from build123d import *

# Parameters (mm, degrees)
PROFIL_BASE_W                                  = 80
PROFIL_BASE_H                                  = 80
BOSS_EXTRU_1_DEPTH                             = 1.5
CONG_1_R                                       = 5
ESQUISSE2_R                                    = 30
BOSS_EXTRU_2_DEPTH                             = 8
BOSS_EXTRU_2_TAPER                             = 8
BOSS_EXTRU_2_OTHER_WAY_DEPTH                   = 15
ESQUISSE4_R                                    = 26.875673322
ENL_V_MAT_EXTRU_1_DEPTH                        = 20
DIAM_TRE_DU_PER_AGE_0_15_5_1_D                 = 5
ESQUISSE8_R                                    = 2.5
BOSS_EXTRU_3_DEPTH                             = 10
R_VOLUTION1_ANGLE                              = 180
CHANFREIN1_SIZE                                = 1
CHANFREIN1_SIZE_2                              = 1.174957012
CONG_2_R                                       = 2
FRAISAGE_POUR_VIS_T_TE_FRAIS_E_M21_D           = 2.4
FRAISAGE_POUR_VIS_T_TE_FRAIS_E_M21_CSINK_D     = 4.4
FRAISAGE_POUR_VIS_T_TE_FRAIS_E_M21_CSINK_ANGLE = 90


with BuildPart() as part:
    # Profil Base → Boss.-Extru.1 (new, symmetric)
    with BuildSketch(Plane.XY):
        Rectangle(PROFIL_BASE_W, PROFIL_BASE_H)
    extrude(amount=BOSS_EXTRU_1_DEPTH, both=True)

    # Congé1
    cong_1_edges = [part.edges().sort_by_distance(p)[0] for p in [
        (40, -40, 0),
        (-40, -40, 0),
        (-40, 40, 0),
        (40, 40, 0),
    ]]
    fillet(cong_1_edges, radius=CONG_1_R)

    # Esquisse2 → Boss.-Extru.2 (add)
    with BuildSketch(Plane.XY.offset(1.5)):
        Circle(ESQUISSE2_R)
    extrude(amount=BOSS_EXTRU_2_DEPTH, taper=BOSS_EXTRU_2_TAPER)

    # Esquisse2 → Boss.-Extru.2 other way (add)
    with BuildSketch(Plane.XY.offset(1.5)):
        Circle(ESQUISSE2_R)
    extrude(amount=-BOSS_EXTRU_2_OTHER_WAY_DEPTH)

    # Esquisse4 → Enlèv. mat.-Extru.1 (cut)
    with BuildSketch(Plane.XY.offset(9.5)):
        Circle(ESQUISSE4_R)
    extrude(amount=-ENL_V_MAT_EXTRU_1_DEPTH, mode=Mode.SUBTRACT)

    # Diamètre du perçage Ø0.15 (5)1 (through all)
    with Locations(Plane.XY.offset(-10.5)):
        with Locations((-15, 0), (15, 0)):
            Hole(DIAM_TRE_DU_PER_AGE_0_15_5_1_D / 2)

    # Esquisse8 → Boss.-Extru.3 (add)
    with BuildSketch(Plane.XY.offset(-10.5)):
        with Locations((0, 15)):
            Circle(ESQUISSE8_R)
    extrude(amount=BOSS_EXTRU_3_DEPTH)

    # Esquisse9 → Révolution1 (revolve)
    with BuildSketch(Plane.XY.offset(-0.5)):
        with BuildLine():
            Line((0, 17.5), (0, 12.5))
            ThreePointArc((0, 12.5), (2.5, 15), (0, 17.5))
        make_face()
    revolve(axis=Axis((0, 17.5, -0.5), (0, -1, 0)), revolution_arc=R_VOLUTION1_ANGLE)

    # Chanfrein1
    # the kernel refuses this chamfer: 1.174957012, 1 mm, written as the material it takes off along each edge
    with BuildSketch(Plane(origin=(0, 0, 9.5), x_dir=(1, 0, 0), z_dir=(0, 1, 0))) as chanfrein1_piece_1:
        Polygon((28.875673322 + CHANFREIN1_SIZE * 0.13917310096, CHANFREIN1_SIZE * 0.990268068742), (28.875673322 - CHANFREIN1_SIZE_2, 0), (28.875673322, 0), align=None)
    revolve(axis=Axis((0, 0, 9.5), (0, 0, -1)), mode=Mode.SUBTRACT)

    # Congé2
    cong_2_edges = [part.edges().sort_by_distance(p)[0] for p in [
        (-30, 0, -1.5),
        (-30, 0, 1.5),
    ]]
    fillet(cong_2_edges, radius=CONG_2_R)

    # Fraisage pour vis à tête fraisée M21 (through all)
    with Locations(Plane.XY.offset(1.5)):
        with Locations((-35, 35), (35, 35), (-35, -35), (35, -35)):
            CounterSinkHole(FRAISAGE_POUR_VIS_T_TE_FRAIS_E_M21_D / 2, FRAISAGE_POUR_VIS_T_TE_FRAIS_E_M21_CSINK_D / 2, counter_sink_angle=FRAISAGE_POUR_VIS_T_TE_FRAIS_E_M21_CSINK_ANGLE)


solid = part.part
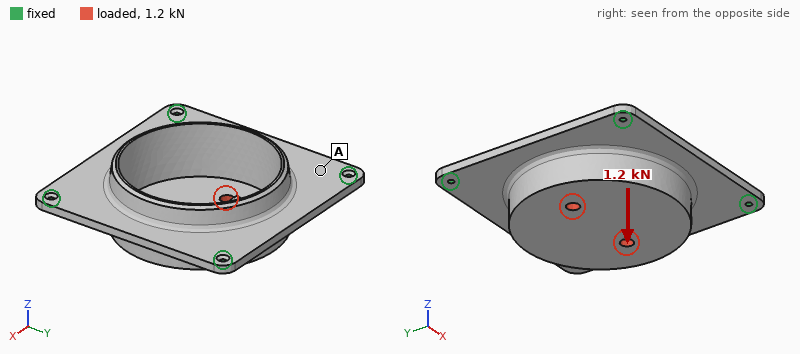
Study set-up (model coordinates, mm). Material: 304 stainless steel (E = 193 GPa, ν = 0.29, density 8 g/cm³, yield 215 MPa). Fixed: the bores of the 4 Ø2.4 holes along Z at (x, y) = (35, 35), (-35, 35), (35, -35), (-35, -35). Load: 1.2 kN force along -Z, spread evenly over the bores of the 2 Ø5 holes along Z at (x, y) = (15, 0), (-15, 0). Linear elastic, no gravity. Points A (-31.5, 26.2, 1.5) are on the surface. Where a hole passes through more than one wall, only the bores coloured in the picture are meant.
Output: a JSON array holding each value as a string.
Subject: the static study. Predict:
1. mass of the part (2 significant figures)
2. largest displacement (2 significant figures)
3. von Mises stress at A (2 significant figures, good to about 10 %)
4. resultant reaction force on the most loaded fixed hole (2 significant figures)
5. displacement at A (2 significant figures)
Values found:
["240 g", "51 µm", "18 MPa", "300 N", "16 µm"]
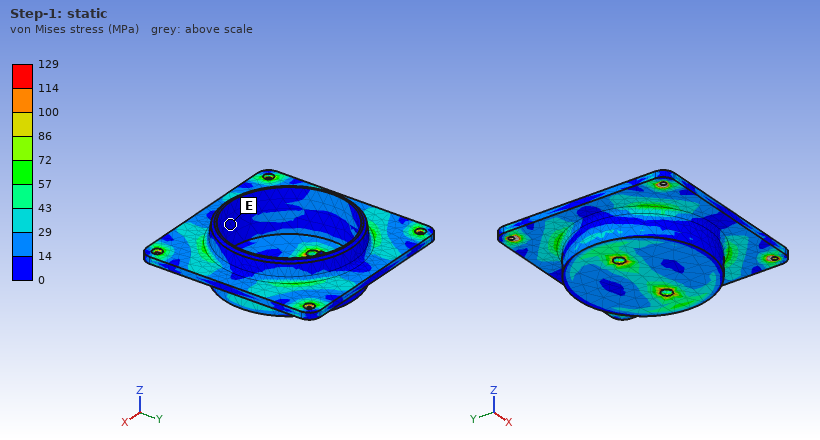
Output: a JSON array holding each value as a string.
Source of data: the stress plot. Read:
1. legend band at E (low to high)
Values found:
["0 to 14 MPa"]
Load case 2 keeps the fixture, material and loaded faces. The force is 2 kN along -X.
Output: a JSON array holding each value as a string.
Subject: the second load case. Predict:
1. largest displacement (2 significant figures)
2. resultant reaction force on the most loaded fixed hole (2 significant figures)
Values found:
["26 µm", "540 N"]
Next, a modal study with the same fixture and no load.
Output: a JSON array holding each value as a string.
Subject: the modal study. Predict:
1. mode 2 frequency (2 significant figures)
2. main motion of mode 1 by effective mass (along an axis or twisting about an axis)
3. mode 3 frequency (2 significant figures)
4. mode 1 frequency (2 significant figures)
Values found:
["3100 Hz", "along Z", "3100 Hz", "2200 Hz"]
